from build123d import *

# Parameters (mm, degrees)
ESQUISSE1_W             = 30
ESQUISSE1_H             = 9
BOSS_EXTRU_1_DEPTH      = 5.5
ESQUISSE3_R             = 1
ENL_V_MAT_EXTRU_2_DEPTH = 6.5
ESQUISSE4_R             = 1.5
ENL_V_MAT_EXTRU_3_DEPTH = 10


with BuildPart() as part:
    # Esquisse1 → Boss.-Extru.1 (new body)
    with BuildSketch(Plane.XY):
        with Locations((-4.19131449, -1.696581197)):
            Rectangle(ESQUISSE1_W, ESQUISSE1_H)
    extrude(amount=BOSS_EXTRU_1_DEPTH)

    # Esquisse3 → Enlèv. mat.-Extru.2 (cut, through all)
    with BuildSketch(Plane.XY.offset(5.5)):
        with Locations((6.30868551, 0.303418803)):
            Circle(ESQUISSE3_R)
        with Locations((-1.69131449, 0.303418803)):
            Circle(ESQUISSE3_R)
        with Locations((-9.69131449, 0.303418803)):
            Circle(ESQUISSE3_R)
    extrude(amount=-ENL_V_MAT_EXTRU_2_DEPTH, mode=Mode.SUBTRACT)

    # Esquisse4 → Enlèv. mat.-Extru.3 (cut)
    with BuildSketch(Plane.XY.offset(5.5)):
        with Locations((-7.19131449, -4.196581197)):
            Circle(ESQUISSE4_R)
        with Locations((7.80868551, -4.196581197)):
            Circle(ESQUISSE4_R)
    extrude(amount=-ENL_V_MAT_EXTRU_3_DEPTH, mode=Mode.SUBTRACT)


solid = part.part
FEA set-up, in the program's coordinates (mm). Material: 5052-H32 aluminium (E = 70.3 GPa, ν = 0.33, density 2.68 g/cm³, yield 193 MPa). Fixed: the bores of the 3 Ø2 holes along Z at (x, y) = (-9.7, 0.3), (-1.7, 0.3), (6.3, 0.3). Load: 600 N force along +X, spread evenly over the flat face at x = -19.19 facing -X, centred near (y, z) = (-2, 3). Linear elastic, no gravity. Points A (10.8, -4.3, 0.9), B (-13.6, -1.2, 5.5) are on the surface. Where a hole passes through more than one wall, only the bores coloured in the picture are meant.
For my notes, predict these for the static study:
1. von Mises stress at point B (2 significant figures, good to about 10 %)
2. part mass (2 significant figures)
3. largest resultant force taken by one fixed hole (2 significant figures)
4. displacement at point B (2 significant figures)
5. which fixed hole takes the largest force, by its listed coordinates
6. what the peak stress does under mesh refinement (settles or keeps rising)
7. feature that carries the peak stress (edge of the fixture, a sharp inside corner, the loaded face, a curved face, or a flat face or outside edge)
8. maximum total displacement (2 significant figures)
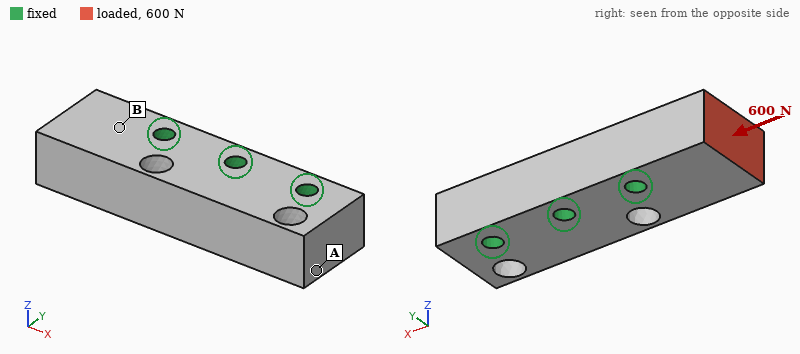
15 MPa
3.6 g
470 N
1.6 µm
(-9.7, 0.3)
keeps rising
edge of the fixture
4.9 µm
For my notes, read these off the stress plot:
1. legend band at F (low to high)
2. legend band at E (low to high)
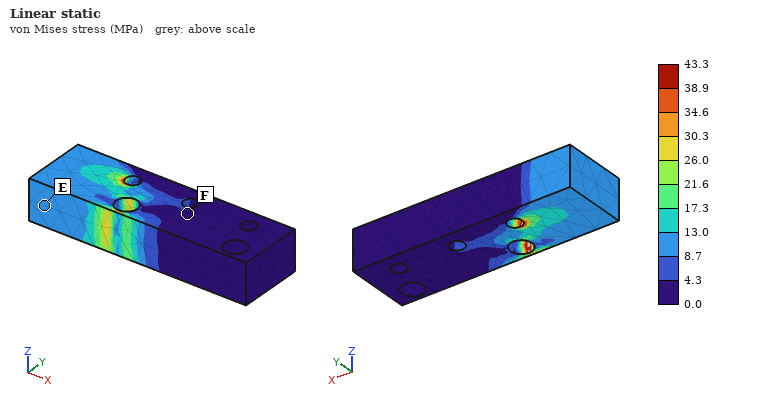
0.0 to 4.3 MPa
8.7 to 13.0 MPa
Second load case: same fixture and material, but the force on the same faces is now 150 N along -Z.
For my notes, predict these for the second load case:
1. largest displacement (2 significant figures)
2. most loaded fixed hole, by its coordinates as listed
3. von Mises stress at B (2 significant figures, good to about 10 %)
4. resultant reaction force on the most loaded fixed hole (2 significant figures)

8.8 µm
(-9.7, 0.3)
20 MPa
180 N
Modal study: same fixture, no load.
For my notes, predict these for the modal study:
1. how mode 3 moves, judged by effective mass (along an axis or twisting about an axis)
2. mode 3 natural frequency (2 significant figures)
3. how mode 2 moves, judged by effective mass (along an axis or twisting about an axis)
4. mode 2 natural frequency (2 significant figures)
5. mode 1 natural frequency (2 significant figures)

twisting about X
59 kHz
along Y
37 kHz
35 kHz
